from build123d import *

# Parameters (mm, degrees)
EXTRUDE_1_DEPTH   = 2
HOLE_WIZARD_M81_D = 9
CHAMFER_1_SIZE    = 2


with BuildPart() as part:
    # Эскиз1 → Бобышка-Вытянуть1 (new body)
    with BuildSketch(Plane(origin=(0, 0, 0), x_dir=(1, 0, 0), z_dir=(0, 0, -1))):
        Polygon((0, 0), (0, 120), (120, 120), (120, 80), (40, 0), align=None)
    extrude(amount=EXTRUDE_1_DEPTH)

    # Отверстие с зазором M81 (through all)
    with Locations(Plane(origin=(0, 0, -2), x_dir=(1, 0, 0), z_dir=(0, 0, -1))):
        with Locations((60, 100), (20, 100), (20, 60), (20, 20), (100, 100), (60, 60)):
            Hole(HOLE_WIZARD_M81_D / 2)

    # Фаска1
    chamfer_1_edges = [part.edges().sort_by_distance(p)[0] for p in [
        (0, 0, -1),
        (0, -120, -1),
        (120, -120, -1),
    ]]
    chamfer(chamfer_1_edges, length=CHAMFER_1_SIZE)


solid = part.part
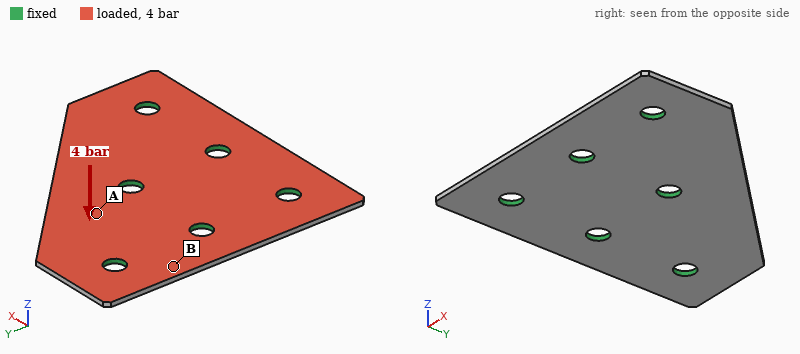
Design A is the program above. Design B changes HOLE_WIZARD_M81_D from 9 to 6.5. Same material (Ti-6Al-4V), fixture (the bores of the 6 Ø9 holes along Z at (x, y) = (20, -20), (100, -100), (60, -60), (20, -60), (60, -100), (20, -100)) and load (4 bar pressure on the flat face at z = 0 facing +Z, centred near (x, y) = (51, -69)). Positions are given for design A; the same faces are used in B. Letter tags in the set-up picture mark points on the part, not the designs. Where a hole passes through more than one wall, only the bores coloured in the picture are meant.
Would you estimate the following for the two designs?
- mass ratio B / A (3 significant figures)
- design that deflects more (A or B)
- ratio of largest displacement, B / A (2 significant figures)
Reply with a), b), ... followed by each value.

a) 1.02
b) B
c) 1.2
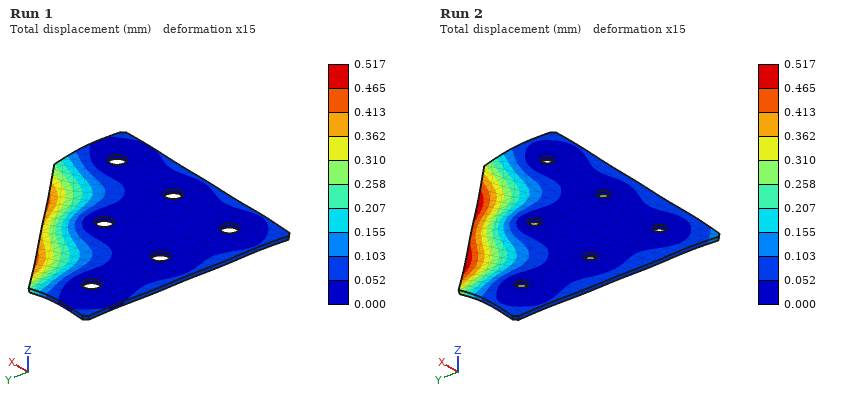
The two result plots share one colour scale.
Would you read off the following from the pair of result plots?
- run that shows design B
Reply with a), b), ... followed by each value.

a) Run 2
